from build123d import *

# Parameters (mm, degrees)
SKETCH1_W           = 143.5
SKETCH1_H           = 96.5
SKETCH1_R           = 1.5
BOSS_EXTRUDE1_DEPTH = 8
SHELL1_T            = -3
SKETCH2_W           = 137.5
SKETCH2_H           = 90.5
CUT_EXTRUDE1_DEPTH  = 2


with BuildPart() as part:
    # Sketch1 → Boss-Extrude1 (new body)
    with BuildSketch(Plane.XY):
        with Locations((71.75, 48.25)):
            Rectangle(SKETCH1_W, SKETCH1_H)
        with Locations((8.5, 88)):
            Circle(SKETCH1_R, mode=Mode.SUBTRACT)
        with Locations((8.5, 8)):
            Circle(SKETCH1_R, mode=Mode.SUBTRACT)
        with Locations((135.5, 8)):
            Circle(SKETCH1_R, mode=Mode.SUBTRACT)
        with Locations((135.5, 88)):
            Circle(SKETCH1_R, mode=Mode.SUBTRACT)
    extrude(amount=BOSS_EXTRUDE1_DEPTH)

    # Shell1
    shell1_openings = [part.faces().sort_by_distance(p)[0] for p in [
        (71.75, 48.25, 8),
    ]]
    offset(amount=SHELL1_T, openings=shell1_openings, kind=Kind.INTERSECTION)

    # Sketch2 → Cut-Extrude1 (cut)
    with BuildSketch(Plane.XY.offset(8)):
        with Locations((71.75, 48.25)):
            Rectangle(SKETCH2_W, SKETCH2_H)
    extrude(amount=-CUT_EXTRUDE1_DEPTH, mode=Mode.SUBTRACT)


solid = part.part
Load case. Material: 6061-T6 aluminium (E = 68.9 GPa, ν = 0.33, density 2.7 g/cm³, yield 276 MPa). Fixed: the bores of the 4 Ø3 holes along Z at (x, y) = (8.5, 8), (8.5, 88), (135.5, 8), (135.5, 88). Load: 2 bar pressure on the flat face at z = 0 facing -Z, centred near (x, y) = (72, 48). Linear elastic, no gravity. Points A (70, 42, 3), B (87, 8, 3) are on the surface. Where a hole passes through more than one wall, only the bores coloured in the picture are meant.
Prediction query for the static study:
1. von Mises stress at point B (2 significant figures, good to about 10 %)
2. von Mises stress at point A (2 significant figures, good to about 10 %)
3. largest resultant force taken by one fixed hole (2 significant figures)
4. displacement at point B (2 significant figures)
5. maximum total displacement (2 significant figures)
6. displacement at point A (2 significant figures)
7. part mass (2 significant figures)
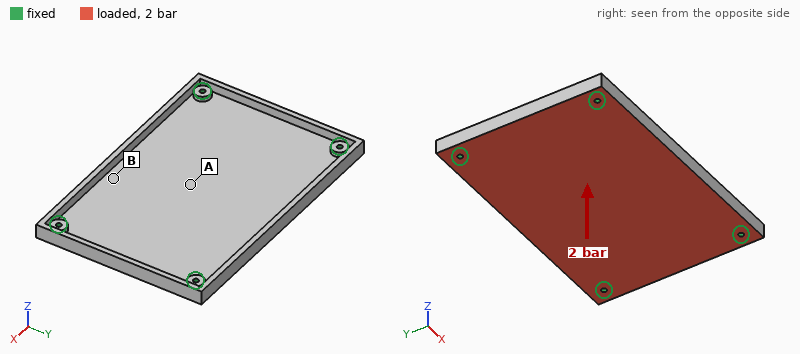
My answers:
25 MPa
62 MPa
740 N
0.40 mm
0.72 mm
0.71 mm
130 g
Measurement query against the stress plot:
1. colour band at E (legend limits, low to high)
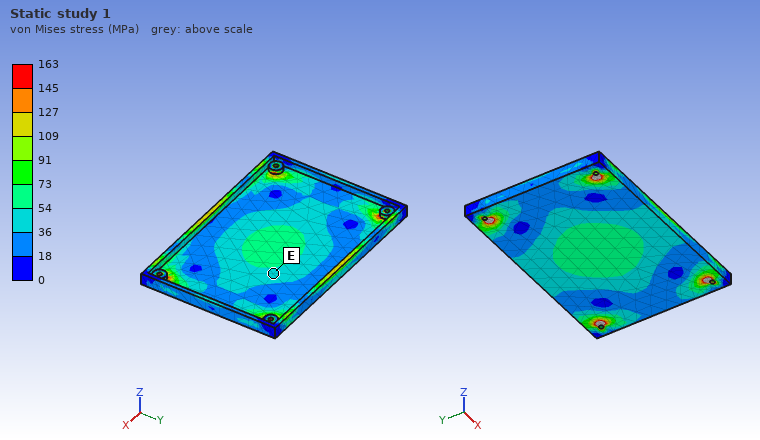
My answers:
36 to 54 MPa
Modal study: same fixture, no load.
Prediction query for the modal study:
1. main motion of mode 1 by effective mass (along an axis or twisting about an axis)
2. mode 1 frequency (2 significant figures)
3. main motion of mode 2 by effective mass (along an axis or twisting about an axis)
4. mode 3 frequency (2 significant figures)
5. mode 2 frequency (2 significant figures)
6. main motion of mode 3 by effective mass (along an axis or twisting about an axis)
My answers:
along Z
1100 Hz
twisting about X
2500 Hz
1800 Hz
twisting about Y
